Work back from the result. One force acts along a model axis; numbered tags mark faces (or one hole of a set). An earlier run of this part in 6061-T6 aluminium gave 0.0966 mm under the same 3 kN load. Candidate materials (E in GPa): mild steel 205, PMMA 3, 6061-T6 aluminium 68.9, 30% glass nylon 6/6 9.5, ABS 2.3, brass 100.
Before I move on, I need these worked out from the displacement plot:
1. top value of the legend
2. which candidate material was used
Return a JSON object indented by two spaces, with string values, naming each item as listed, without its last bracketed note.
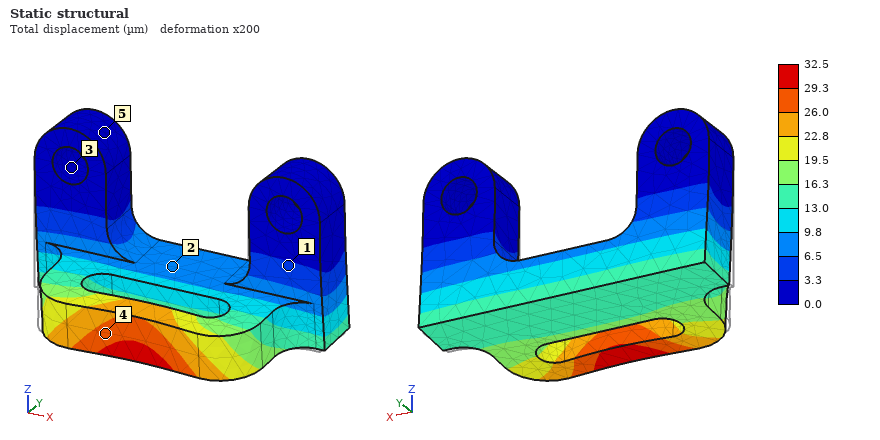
{
  "top value of the legend": "32.5 µm",
  "which candidate material was used": "mild steel"
}
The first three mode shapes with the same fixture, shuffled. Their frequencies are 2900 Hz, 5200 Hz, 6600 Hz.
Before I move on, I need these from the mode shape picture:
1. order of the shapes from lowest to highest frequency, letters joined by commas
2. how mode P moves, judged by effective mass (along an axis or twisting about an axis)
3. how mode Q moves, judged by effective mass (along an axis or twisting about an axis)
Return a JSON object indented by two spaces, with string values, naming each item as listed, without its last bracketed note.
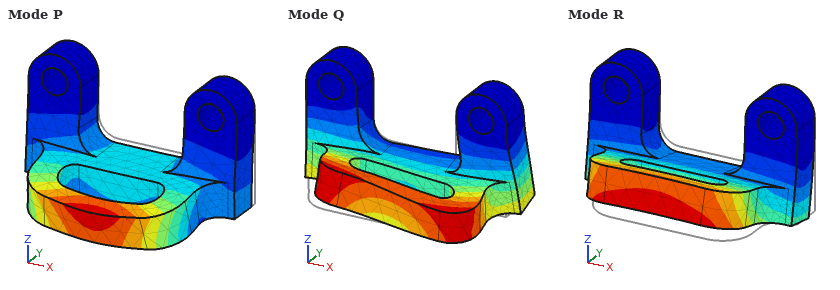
{
  "order of the shapes from lowest to highest frequency, letters joined by commas": "R, Q, P",
  "how mode P moves, judged by effective mass": "along Y",
  "how mode Q moves, judged by effective mass": "along X"
}
